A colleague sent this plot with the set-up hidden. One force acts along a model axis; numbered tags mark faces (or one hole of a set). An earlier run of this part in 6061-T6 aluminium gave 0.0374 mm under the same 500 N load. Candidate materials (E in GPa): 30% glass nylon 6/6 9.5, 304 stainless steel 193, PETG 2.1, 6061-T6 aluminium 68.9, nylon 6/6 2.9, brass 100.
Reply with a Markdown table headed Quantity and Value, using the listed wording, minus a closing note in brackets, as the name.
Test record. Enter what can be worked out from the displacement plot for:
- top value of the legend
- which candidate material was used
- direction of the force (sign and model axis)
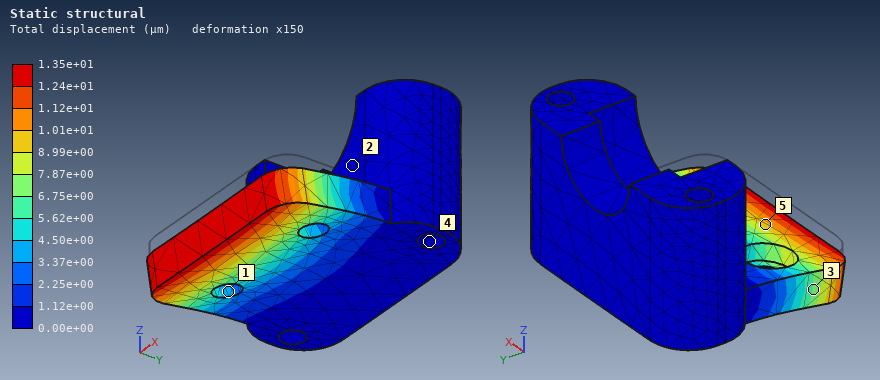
| Quantity | Value |
|---|---|
| top value of the legend | 1.35e+01 µm |
| which candidate material was used | 304 stainless steel |
| direction of the force | -Z |
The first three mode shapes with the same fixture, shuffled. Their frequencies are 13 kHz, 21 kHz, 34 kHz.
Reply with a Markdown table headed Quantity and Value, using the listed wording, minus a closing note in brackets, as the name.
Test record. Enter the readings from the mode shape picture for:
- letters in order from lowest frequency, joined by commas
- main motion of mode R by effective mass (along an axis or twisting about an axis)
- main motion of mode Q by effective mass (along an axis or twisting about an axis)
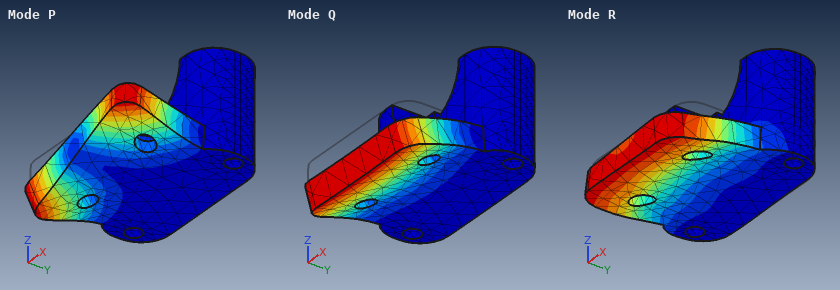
| Quantity | Value |
|---|---|
| letters in order from lowest frequency, joined by commas | Q, P, R |
| main motion of mode R by effective mass | along X |
| main motion of mode Q by effective mass | along Z |
